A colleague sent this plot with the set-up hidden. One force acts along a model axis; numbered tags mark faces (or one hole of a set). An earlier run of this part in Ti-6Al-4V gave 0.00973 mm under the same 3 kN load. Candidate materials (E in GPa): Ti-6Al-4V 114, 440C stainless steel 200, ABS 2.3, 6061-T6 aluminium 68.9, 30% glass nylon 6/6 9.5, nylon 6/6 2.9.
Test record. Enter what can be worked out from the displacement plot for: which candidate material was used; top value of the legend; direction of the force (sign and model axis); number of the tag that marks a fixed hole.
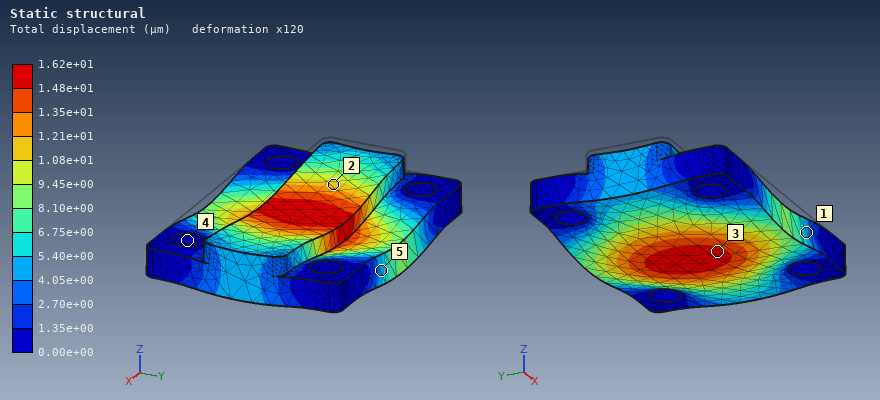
6061-T6 aluminium
1.62e+01 µm
-Z
4
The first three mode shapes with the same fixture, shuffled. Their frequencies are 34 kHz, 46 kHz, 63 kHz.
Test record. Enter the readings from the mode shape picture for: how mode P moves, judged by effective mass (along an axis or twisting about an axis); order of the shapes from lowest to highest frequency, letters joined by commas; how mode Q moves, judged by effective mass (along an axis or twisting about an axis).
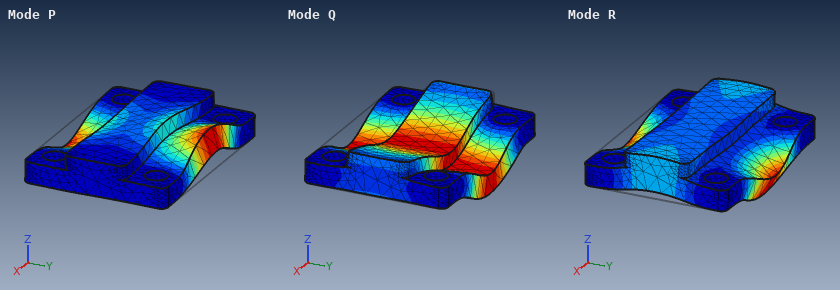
twisting about X
Q, P, R
along Z
